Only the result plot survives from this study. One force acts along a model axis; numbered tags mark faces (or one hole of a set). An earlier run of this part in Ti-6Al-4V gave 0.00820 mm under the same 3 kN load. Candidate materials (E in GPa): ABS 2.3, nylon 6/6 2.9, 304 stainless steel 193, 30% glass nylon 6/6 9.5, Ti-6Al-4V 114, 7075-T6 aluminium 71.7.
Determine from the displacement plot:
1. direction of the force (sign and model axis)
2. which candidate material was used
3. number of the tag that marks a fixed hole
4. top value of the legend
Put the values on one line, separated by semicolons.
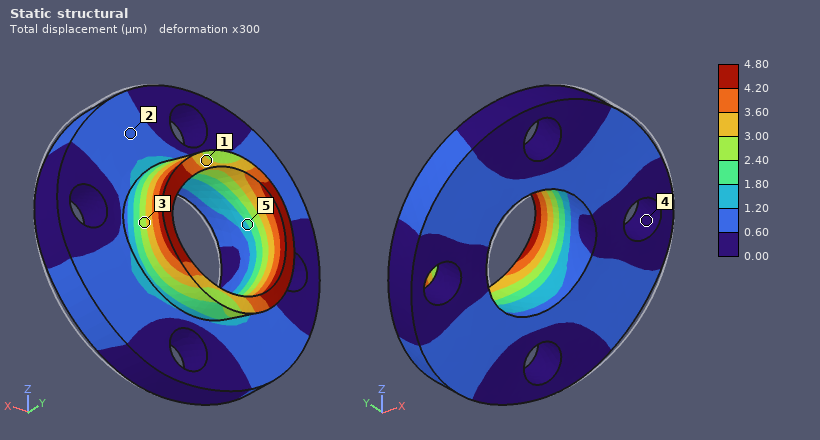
-X; 304 stainless steel; 4; 4.80 µm
